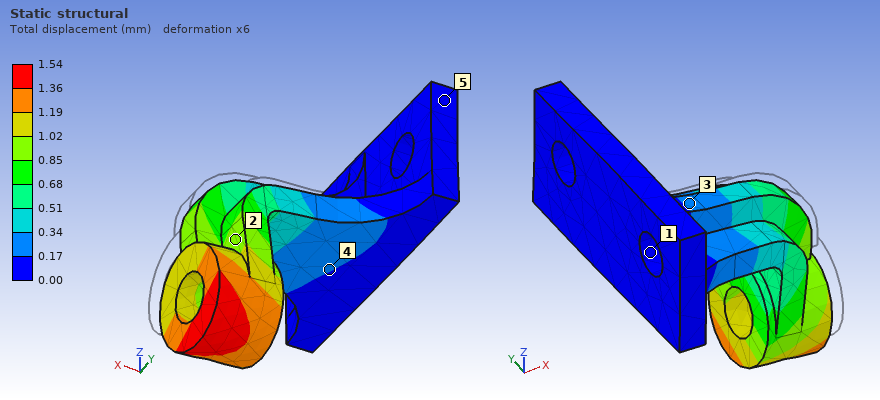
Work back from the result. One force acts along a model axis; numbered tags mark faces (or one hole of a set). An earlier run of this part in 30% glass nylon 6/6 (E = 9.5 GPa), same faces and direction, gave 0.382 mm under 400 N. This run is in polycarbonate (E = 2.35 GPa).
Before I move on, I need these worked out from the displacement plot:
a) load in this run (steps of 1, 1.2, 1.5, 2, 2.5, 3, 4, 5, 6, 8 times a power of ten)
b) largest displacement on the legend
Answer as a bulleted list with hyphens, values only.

- 400 N
- 1.54 mm
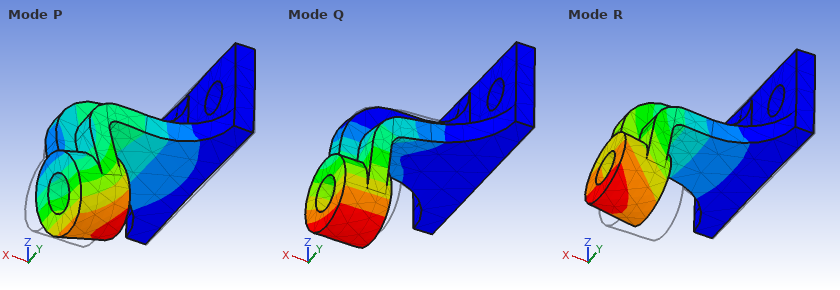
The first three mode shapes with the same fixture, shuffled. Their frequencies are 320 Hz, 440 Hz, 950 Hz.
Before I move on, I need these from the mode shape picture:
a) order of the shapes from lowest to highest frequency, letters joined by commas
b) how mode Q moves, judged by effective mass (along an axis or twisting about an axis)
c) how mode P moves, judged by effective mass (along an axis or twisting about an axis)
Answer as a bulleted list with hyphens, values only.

- R, Q, P
- along Y
- along Z
